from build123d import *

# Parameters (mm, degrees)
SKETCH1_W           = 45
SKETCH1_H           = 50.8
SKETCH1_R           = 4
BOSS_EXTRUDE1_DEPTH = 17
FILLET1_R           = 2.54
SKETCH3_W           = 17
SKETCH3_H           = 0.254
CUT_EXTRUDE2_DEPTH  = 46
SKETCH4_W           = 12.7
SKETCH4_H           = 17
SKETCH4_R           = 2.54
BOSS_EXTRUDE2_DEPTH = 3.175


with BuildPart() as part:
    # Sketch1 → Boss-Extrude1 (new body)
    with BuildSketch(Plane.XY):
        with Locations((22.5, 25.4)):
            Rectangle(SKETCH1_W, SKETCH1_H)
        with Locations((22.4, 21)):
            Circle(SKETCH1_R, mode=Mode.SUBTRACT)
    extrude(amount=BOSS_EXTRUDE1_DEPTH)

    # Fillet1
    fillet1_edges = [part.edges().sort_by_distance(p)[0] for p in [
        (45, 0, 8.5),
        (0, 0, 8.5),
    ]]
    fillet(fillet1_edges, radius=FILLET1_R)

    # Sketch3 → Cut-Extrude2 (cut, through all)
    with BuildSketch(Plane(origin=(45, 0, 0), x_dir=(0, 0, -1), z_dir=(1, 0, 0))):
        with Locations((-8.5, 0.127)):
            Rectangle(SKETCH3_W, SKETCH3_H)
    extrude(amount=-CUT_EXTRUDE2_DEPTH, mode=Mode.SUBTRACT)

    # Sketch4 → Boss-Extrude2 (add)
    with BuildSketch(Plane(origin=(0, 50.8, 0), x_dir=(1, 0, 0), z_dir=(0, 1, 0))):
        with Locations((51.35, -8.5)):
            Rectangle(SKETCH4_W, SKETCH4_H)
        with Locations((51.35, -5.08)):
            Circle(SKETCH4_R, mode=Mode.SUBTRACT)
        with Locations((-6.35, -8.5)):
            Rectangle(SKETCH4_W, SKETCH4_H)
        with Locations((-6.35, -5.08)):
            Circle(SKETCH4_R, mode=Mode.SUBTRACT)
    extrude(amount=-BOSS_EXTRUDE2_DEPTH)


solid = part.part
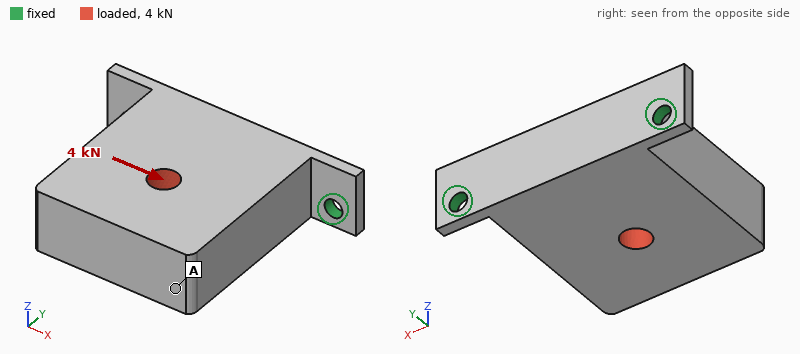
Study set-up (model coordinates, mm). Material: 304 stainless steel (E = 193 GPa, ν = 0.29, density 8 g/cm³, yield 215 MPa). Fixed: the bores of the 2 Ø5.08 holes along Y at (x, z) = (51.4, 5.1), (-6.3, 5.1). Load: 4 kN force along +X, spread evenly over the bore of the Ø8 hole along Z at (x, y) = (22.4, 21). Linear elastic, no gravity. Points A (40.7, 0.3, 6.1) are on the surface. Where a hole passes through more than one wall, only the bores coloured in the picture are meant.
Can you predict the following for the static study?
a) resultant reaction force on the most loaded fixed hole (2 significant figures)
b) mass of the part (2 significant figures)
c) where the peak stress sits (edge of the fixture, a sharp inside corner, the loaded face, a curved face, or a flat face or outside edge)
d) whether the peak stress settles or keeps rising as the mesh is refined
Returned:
3.0 kN
310 g
edge of the fixture
keeps rising
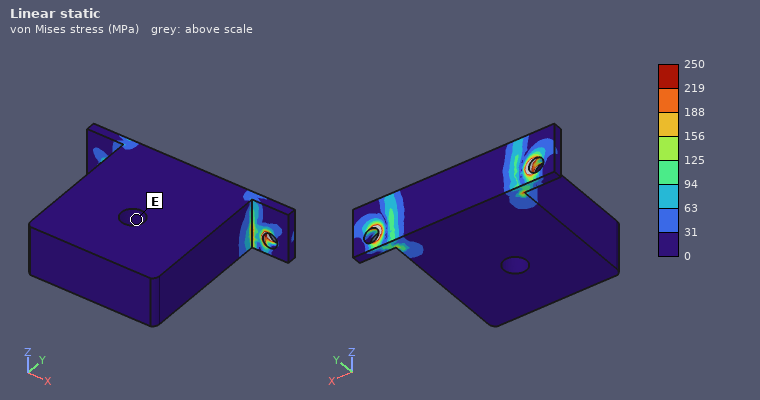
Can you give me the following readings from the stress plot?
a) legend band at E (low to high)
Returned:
0 to 31 MPa
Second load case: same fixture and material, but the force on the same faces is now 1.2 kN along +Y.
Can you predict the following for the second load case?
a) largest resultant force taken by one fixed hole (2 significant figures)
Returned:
670 N
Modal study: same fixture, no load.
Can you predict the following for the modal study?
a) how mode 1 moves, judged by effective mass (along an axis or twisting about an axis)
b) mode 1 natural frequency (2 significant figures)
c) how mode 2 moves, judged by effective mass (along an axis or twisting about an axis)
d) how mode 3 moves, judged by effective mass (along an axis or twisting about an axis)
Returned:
along Z
740 Hz
along X
along Y
